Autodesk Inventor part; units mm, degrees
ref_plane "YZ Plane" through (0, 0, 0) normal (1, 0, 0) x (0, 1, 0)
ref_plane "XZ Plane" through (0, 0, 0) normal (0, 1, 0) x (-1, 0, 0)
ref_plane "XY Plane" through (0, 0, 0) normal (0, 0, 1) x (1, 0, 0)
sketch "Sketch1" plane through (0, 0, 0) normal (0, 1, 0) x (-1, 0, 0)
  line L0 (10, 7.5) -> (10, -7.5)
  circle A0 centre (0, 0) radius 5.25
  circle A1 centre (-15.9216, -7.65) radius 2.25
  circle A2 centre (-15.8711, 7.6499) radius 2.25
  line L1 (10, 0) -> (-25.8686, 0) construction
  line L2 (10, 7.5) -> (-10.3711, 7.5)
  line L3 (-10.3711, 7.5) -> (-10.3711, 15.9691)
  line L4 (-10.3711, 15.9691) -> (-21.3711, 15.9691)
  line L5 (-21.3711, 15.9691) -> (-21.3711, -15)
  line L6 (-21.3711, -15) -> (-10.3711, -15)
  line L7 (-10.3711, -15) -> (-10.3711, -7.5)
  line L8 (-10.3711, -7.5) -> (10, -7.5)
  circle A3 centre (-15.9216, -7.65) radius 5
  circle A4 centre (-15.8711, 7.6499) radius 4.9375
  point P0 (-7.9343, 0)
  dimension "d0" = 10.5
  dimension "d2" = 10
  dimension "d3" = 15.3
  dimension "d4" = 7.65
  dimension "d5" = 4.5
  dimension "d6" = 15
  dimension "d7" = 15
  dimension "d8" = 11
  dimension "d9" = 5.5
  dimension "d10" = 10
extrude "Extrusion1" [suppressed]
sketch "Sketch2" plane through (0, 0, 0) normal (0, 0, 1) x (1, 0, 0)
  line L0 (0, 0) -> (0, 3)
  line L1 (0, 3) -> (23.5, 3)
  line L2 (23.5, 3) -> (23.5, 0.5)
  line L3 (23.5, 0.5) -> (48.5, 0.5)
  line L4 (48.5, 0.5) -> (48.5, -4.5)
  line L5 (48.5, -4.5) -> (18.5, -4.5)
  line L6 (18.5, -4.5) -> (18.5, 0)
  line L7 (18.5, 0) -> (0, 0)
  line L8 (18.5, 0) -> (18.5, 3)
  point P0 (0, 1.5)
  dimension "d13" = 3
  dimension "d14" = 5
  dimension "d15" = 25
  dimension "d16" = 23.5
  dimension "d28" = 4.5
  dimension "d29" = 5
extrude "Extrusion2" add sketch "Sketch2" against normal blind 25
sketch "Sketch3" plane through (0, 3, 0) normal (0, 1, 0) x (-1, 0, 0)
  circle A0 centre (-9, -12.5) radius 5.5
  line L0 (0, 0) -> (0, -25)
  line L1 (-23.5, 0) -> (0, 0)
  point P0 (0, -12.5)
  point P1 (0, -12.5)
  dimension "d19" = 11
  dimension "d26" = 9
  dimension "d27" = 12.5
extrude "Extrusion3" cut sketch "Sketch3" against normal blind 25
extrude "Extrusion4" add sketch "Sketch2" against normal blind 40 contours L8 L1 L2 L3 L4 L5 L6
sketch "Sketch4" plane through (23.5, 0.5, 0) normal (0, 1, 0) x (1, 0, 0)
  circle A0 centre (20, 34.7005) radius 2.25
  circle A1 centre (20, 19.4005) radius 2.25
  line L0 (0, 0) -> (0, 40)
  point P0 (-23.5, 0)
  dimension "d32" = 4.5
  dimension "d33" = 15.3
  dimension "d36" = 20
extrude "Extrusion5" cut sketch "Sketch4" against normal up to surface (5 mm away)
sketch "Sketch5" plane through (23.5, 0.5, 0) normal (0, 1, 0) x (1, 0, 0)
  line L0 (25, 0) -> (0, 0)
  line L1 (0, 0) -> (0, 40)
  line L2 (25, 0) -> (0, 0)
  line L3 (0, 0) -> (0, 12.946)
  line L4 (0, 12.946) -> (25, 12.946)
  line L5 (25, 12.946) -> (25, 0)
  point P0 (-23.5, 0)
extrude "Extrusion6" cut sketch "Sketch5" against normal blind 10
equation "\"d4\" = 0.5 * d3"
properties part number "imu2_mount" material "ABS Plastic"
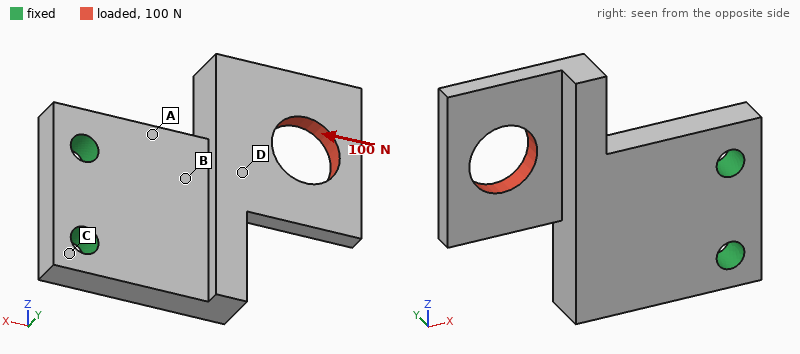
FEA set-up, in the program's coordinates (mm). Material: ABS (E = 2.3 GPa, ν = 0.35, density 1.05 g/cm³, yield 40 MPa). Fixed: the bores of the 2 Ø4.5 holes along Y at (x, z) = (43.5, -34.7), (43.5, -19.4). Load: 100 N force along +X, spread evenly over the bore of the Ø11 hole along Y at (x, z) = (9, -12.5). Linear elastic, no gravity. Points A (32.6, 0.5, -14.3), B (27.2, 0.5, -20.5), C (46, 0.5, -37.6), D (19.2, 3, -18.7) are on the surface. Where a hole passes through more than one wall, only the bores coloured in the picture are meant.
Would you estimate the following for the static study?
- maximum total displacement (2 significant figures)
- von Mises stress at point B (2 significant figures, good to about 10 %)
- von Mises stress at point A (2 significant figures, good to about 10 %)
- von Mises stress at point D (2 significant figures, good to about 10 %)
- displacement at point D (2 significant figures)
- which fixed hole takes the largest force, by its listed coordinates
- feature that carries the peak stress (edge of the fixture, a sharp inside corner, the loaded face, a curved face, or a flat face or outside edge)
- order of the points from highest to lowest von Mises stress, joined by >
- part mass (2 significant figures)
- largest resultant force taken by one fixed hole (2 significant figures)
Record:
0.64 mm
5.2 MPa
7.1 MPa
3.7 MPa
0.19 mm
(43.5, -19.4)
a flat face or outside edge
A > B > D > C
6.1 g
130 N
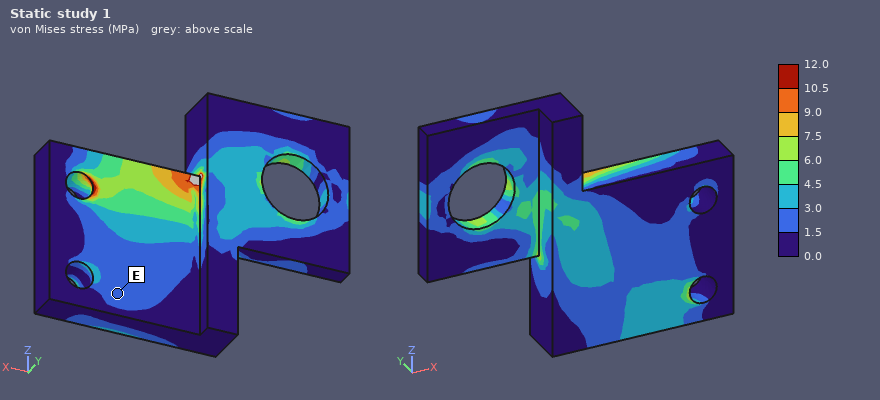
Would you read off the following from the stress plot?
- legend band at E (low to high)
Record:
1.5 to 3.0 MPa
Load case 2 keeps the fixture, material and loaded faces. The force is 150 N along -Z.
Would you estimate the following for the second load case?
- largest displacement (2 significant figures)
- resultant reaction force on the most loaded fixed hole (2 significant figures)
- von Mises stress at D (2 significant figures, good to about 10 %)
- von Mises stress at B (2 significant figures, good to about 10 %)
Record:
0.67 mm
300 N
7.0 MPa
2.2 MPa
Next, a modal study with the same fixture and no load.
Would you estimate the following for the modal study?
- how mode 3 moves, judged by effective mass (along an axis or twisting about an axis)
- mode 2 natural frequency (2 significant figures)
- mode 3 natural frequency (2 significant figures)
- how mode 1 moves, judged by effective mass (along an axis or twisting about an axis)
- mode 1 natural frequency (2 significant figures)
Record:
along Z
1900 Hz
2200 Hz
along Y
730 Hz
